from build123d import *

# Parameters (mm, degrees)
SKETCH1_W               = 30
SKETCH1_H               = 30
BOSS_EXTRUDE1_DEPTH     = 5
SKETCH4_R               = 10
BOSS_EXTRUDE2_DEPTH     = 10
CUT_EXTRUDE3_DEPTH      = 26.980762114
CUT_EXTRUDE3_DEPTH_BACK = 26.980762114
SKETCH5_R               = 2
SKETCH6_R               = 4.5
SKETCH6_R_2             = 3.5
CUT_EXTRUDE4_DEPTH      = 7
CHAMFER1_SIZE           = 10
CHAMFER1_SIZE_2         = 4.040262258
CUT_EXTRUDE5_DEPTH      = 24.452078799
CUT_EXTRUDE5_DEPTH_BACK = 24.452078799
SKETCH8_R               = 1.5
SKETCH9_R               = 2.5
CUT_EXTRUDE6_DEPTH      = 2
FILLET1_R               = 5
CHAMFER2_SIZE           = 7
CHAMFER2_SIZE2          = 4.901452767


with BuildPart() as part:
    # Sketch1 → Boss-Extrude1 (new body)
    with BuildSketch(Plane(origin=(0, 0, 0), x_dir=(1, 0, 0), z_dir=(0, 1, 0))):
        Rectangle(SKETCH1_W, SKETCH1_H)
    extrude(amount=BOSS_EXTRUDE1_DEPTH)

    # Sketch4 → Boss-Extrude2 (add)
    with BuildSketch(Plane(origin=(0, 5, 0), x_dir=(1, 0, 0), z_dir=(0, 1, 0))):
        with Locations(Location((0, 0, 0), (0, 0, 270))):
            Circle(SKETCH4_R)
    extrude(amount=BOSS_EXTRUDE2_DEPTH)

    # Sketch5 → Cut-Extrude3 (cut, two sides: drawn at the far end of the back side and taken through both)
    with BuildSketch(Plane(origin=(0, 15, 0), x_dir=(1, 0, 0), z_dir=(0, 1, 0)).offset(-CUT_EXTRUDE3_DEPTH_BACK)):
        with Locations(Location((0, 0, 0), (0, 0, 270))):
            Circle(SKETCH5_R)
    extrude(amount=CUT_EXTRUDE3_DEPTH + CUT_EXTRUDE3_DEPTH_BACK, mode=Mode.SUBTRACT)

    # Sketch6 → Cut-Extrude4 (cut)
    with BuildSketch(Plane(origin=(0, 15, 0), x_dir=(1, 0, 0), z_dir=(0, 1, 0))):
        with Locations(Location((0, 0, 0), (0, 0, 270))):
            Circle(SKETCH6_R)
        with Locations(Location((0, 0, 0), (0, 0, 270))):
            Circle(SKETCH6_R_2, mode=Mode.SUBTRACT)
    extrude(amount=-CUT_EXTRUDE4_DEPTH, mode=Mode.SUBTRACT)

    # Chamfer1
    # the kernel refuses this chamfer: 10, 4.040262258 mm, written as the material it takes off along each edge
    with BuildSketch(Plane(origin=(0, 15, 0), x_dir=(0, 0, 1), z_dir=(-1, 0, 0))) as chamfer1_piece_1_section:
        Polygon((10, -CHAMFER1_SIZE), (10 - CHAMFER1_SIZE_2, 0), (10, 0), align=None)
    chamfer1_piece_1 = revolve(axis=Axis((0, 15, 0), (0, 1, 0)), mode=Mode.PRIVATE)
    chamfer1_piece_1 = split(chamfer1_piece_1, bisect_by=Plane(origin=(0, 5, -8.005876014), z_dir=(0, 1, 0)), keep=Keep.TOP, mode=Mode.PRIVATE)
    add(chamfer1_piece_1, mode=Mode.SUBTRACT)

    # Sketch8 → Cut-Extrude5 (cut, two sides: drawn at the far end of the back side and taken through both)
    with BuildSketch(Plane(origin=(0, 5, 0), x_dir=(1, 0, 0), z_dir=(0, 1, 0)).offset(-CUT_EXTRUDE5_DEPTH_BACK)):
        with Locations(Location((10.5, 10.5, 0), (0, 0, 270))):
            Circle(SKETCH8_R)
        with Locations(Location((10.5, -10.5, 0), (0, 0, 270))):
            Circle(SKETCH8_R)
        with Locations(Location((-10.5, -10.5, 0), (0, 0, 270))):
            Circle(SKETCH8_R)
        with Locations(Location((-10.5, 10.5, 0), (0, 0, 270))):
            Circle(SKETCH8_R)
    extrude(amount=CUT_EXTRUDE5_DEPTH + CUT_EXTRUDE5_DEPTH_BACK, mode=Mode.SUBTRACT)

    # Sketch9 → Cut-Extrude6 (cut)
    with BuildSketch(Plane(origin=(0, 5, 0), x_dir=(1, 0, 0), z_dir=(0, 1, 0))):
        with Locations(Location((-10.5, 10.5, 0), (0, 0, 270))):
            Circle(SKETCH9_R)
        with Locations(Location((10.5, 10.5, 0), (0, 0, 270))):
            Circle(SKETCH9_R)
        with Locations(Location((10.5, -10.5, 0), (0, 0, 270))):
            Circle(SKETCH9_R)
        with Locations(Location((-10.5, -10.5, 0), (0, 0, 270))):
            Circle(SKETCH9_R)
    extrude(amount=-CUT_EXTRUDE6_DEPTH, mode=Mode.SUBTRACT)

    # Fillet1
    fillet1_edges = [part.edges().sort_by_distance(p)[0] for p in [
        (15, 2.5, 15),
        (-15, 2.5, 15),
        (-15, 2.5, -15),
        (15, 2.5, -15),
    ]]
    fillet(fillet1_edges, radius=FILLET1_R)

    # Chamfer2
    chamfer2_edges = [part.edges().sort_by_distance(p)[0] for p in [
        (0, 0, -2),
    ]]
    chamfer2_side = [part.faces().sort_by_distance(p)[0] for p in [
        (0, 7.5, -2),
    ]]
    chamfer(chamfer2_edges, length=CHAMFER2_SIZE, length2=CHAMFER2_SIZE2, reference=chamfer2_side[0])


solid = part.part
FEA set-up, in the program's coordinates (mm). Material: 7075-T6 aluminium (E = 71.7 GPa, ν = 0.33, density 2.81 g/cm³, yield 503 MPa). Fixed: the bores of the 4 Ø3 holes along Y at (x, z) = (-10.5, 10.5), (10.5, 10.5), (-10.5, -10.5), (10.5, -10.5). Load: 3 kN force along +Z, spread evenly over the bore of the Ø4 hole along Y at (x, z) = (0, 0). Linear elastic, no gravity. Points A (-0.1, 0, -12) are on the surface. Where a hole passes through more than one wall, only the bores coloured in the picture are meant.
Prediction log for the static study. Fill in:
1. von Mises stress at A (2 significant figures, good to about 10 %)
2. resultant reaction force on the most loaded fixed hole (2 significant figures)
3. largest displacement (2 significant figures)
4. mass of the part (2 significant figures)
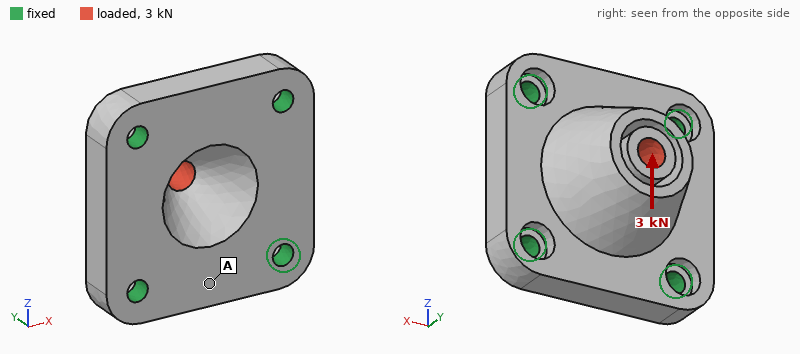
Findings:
28 MPa
1.2 kN
74 µm
15 g
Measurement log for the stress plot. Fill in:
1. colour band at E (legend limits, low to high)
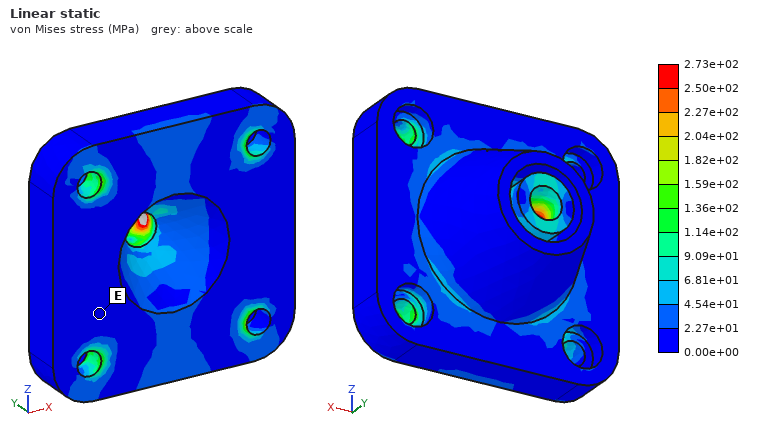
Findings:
0.00e+00 to 2.27e+01 MPa
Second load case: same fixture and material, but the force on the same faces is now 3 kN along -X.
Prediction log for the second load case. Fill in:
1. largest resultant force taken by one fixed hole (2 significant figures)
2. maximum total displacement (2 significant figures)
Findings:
1.2 kN
74 µm
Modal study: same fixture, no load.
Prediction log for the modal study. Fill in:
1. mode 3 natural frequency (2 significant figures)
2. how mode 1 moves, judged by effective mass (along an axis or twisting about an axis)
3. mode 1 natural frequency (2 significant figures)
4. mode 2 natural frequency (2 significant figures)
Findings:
33 kHz
along Y
29 kHz
33 kHz
